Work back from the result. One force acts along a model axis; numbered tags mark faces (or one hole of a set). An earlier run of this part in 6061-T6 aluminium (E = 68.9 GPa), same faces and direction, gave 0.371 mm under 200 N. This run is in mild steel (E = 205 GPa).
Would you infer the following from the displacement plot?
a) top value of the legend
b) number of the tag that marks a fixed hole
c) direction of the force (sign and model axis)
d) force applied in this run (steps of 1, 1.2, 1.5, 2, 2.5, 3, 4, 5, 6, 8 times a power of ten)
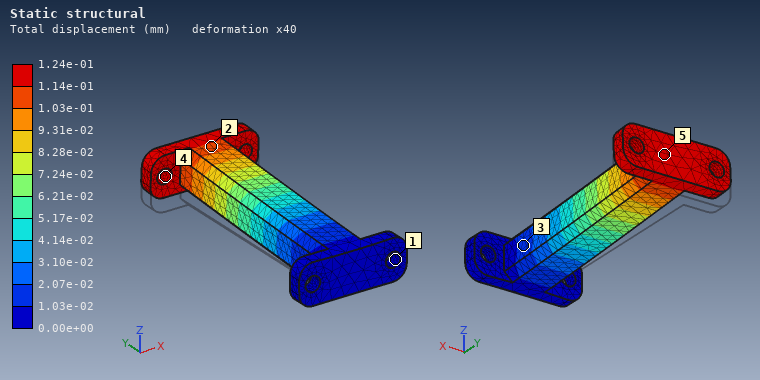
1.24e-01 mm
1
+Z
200 N
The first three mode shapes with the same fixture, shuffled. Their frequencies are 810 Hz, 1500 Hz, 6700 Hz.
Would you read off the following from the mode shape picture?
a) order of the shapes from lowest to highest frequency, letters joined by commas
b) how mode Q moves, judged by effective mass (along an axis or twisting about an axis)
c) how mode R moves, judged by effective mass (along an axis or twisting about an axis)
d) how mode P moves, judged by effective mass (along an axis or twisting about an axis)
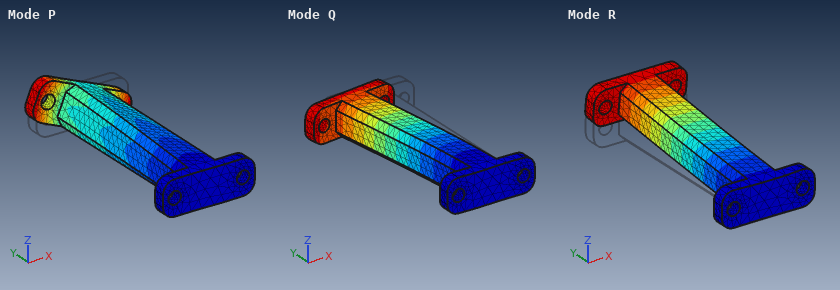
R, Q, P
along X
along Z
twisting about Y
